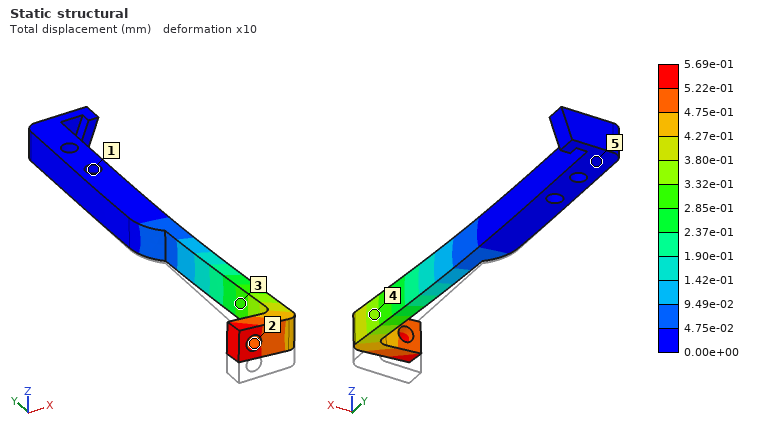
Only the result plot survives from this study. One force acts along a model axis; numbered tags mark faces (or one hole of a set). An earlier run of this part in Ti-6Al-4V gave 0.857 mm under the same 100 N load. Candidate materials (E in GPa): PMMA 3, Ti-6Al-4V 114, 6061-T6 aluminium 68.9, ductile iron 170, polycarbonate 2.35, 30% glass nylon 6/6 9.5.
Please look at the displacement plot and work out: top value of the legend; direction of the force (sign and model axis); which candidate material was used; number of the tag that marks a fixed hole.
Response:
5.69e-01 mm
+Z
ductile iron
1
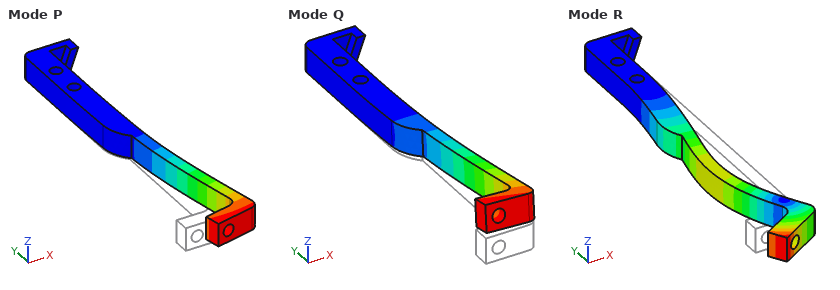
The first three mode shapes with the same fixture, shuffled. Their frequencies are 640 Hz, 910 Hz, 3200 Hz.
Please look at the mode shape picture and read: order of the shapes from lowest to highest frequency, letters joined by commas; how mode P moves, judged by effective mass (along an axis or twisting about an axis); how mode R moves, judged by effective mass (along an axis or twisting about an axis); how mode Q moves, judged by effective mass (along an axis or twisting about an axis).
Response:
P, Q, R
along X
along X
along Z
